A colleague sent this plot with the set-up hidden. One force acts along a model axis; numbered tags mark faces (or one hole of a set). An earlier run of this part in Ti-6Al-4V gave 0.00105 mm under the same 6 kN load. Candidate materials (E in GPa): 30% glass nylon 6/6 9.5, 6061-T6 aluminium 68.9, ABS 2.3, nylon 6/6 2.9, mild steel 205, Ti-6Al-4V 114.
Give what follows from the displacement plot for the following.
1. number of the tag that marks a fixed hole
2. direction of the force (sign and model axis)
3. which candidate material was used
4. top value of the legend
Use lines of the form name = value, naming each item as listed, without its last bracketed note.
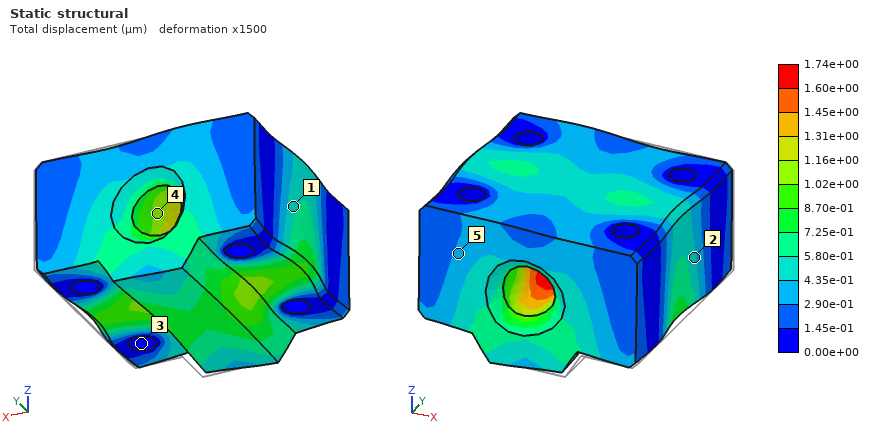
number of the tag that marks a fixed hole = 3
direction of the force = -X
which candidate material was used = 6061-T6 aluminium
top value of the legend = 1.74e+00 µm
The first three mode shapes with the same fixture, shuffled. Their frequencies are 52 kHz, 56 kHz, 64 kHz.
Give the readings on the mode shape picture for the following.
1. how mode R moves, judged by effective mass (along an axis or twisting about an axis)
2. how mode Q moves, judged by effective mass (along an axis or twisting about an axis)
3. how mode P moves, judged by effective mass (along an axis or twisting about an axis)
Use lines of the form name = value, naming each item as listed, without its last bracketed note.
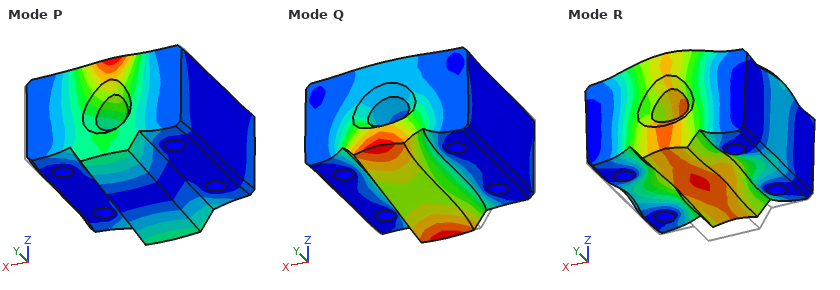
how mode R moves, judged by effective mass = along Z
how mode Q moves, judged by effective mass = along Y
how mode P moves, judged by effective mass = along Y
